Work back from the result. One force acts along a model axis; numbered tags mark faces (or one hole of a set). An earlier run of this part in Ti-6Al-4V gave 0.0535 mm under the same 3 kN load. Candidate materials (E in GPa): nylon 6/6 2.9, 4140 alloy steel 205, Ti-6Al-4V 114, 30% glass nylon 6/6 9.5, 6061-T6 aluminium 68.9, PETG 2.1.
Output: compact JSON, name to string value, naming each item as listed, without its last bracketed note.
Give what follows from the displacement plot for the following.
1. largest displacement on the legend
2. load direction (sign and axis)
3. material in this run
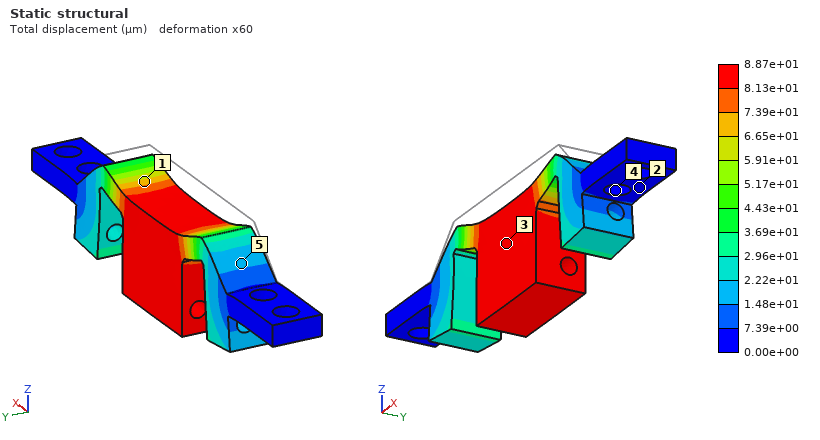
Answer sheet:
{"largest displacement on the legend": "8.87e+01 µm", "load direction": "-Z", "material in this run": "6061-T6 aluminium"}
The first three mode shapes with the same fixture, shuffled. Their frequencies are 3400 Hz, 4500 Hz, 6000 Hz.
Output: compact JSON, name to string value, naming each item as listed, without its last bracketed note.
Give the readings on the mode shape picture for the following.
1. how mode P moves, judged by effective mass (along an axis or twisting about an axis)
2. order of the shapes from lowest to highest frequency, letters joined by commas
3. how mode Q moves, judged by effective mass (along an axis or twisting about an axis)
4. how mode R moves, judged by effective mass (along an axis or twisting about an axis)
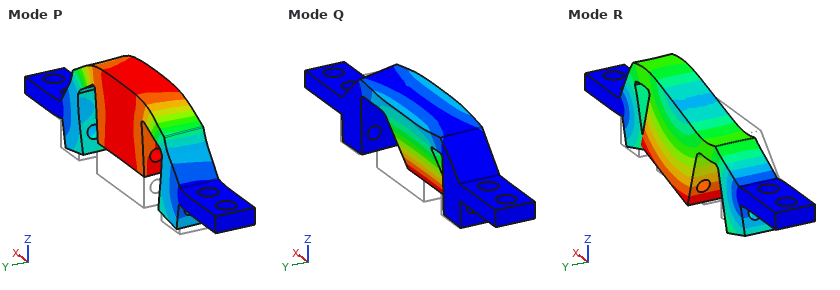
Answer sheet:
{"how mode P moves, judged by effective mass": "along Z", "order of the shapes from lowest to highest frequency, letters joined by commas": "Q, R, P", "how mode Q moves, judged by effective mass": "along Y", "how mode R moves, judged by effective mass": "along X"}
